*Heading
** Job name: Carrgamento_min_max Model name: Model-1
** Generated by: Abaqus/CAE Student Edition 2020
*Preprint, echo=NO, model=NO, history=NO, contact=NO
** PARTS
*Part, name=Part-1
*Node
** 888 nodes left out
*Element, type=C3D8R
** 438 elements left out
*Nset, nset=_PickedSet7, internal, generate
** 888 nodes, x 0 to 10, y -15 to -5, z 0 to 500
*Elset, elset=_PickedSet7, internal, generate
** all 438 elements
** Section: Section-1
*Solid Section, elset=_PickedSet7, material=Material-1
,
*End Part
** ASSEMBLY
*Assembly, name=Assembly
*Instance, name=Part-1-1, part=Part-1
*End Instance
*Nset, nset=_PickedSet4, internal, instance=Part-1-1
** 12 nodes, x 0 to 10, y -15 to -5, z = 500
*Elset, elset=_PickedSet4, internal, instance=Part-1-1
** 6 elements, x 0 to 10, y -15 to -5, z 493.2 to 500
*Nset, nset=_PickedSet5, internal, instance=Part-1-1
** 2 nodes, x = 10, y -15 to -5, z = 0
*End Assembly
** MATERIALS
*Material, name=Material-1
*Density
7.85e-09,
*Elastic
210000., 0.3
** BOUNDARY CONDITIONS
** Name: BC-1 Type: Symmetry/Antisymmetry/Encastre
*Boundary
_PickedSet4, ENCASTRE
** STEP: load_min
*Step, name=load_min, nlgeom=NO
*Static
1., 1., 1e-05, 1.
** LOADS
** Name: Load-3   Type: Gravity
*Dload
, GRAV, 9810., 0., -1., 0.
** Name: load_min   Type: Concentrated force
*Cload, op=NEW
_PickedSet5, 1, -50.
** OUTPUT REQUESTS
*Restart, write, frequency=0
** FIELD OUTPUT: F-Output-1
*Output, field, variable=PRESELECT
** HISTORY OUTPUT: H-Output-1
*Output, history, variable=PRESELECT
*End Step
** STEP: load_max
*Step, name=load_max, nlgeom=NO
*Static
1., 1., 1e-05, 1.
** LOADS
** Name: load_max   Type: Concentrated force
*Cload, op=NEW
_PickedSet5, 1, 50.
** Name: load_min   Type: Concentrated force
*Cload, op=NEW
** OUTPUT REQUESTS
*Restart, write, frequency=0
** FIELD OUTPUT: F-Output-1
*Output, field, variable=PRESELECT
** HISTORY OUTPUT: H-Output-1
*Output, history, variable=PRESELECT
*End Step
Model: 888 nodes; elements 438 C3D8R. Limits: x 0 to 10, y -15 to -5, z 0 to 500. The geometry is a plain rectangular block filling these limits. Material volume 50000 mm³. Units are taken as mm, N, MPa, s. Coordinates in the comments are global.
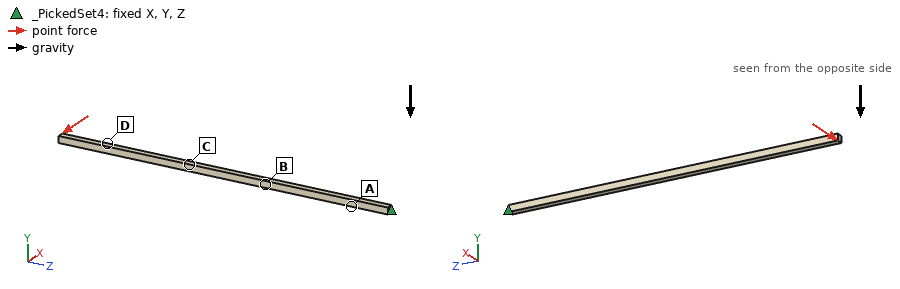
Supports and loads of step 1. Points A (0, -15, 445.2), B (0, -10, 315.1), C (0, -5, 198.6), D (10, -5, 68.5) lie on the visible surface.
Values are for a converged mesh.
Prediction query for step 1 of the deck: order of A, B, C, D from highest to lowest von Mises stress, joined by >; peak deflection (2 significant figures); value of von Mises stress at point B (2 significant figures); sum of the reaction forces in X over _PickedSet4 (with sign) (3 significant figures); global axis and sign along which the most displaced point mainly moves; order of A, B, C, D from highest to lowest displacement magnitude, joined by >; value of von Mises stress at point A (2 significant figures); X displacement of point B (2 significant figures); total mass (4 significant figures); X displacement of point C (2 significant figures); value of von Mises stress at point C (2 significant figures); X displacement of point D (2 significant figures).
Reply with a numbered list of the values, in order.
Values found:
1. A > B > C > D
2. 24 mm
3. 190 MPa
4. 100 N
5. -X
6. D > C > B > A
7. 270 MPa
8. -4.3 mm
9. 0.3925 kg
10. -10 mm
11. 120 MPa
12. -19 mm
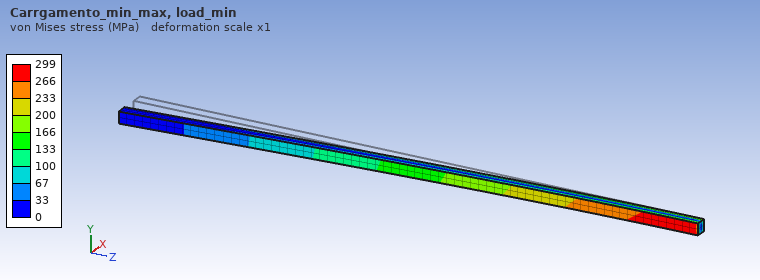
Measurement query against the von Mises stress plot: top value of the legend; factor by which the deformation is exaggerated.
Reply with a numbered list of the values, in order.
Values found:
1. 299 MPa
2. 1
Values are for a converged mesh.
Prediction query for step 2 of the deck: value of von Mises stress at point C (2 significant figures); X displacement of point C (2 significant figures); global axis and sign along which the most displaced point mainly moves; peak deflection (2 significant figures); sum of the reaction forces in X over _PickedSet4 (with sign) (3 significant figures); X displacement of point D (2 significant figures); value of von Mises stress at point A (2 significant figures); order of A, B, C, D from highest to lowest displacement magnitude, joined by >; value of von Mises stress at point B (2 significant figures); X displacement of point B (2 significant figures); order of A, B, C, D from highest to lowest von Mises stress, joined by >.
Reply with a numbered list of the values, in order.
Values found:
1. 120 MPa
2. 10 mm
3. +X
4. 24 mm
5. -100 N
6. 19 mm
7. 260 MPa
8. D > C > B > A
9. 190 MPa
10. 4.3 mm
11. A > B > C > D
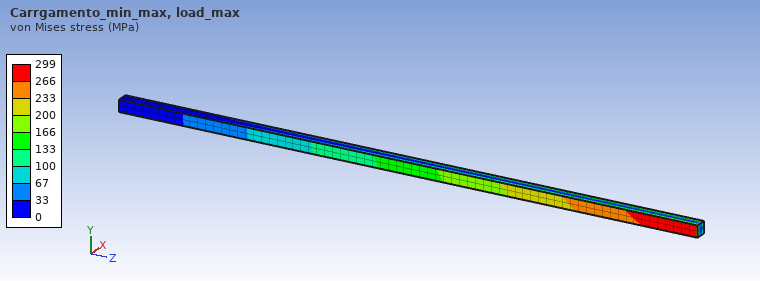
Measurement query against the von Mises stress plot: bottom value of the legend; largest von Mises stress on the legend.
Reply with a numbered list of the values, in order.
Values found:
1. 0 MPa
2. 299 MPa
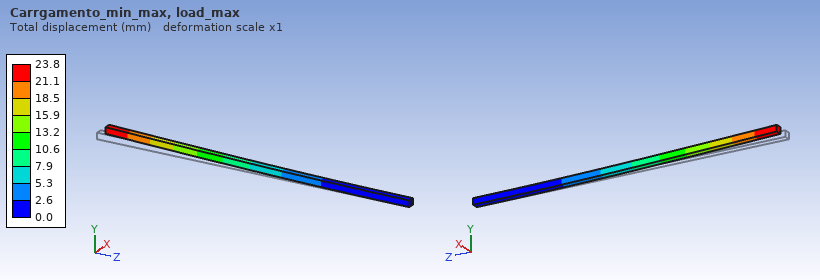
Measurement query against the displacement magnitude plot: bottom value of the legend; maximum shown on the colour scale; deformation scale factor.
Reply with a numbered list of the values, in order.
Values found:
1. 0.0 mm
2. 23.8 mm
3. 1
